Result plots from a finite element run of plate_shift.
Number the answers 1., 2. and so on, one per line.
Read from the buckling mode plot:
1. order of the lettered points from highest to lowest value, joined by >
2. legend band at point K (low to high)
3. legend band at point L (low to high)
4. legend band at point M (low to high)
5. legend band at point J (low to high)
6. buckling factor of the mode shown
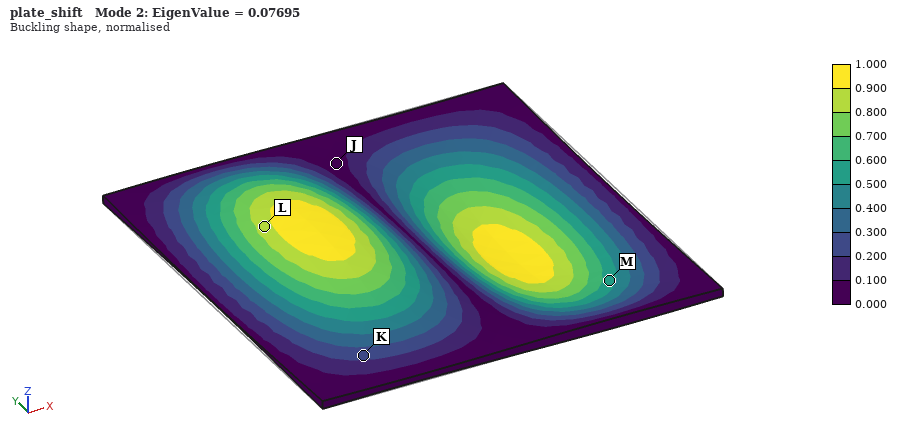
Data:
1. L > M > K > J
2. 0.200 to 0.300
3. 0.800 to 0.900
4. 0.500 to 0.600
5. 0.000 to 0.100
6. 0.07695
